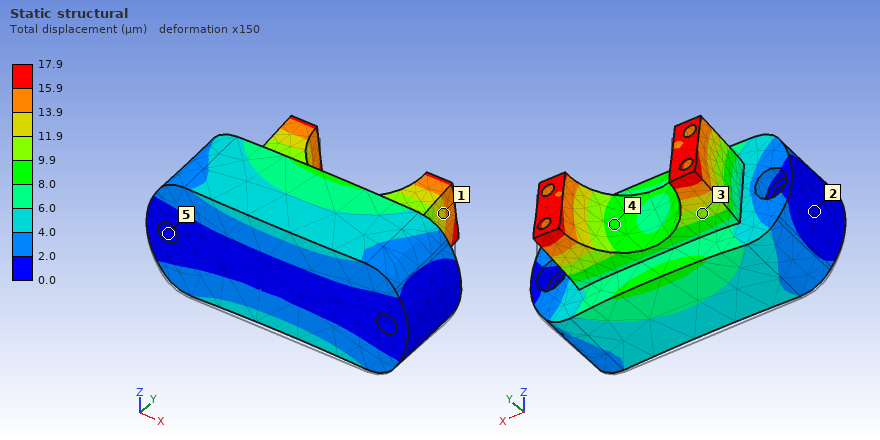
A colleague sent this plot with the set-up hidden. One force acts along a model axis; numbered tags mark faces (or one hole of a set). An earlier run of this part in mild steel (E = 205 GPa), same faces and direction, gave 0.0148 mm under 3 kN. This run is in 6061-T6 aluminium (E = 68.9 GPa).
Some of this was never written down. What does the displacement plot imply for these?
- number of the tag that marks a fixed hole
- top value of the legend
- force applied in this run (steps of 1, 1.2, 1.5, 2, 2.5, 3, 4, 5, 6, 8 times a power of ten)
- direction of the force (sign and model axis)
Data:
5
17.9 µm
1.2 kN
+Z
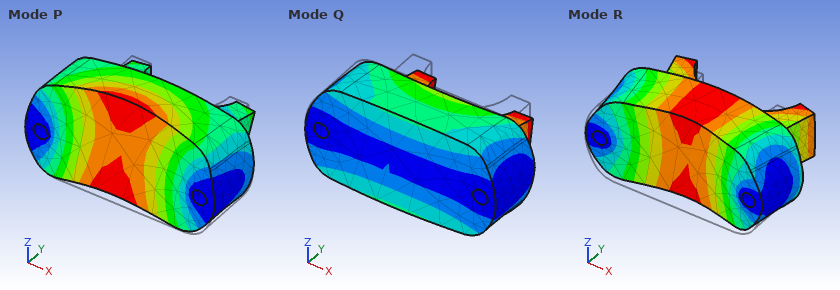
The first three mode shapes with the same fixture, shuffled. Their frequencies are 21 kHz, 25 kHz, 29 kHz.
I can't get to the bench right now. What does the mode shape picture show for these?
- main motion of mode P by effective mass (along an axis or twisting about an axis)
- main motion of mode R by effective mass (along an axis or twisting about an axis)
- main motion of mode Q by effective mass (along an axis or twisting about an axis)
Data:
along Z
along Y
along Z
